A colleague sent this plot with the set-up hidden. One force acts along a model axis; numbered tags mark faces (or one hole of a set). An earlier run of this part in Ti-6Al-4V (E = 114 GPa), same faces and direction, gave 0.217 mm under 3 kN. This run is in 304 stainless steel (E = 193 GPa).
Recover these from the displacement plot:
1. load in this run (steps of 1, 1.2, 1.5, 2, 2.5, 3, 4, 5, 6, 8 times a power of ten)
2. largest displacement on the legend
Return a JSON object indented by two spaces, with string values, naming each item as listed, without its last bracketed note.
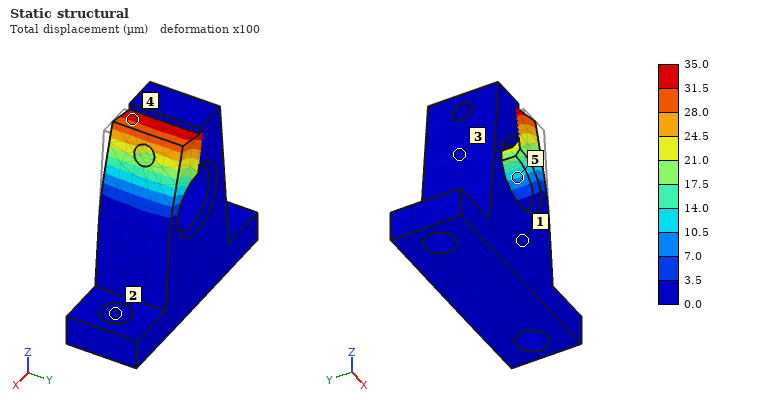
{
  "load in this run": "800 N",
  "largest displacement on the legend": "35.0 µm"
}
